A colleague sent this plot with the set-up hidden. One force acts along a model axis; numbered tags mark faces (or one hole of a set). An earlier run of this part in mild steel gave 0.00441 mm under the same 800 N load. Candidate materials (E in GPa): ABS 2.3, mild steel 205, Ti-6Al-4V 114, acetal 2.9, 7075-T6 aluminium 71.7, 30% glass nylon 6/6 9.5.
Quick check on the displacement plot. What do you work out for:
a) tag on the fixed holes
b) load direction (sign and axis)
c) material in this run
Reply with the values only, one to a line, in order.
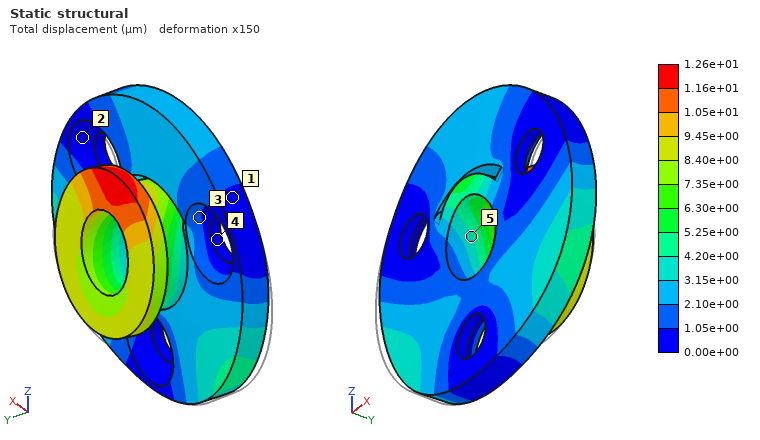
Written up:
4
+Z
7075-T6 aluminium
